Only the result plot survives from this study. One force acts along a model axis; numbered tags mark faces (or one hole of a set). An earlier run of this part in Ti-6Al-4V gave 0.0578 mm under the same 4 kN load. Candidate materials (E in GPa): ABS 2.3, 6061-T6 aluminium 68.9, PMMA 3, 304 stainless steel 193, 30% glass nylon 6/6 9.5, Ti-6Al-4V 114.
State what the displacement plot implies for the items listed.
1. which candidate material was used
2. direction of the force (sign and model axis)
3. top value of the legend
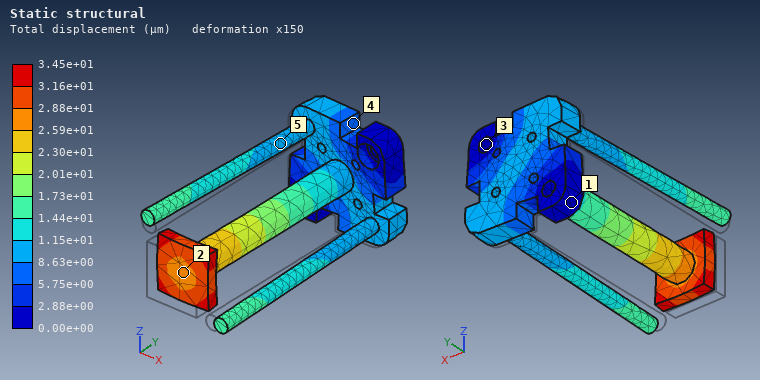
304 stainless steel
+Y
3.45e+01 µm
